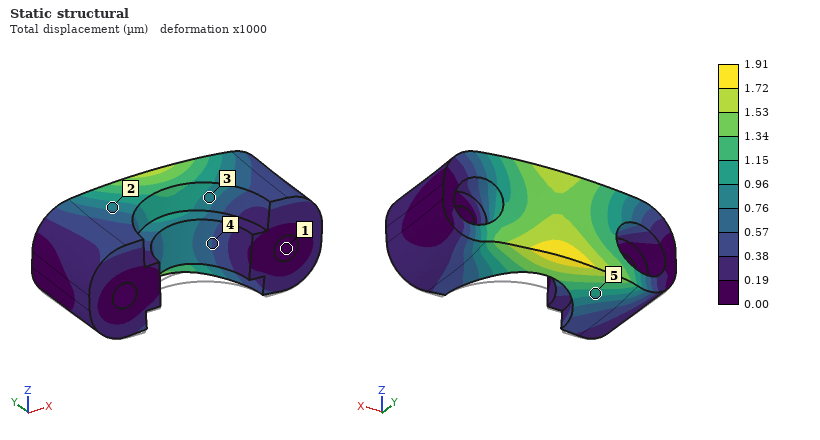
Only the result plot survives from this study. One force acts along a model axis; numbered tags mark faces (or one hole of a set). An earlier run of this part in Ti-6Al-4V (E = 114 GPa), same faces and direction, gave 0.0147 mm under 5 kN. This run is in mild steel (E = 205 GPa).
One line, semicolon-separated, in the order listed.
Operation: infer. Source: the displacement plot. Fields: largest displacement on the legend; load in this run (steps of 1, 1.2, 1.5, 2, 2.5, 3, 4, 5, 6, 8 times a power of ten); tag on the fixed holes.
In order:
1.91 µm; 1.2 kN; 1
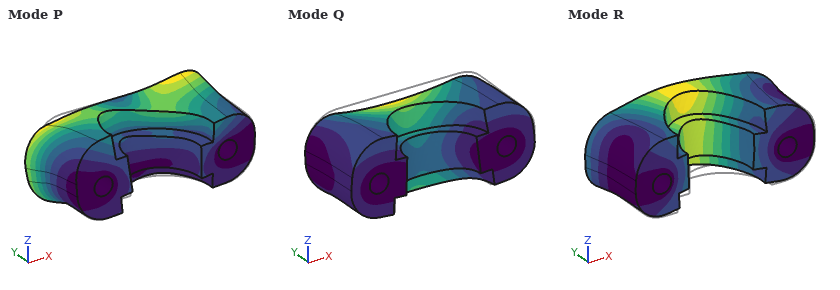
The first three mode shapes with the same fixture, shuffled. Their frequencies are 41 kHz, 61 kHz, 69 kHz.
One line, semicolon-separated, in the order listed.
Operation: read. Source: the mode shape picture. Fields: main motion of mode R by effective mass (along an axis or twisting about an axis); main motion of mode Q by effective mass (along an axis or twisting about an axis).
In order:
along Y; along Z
